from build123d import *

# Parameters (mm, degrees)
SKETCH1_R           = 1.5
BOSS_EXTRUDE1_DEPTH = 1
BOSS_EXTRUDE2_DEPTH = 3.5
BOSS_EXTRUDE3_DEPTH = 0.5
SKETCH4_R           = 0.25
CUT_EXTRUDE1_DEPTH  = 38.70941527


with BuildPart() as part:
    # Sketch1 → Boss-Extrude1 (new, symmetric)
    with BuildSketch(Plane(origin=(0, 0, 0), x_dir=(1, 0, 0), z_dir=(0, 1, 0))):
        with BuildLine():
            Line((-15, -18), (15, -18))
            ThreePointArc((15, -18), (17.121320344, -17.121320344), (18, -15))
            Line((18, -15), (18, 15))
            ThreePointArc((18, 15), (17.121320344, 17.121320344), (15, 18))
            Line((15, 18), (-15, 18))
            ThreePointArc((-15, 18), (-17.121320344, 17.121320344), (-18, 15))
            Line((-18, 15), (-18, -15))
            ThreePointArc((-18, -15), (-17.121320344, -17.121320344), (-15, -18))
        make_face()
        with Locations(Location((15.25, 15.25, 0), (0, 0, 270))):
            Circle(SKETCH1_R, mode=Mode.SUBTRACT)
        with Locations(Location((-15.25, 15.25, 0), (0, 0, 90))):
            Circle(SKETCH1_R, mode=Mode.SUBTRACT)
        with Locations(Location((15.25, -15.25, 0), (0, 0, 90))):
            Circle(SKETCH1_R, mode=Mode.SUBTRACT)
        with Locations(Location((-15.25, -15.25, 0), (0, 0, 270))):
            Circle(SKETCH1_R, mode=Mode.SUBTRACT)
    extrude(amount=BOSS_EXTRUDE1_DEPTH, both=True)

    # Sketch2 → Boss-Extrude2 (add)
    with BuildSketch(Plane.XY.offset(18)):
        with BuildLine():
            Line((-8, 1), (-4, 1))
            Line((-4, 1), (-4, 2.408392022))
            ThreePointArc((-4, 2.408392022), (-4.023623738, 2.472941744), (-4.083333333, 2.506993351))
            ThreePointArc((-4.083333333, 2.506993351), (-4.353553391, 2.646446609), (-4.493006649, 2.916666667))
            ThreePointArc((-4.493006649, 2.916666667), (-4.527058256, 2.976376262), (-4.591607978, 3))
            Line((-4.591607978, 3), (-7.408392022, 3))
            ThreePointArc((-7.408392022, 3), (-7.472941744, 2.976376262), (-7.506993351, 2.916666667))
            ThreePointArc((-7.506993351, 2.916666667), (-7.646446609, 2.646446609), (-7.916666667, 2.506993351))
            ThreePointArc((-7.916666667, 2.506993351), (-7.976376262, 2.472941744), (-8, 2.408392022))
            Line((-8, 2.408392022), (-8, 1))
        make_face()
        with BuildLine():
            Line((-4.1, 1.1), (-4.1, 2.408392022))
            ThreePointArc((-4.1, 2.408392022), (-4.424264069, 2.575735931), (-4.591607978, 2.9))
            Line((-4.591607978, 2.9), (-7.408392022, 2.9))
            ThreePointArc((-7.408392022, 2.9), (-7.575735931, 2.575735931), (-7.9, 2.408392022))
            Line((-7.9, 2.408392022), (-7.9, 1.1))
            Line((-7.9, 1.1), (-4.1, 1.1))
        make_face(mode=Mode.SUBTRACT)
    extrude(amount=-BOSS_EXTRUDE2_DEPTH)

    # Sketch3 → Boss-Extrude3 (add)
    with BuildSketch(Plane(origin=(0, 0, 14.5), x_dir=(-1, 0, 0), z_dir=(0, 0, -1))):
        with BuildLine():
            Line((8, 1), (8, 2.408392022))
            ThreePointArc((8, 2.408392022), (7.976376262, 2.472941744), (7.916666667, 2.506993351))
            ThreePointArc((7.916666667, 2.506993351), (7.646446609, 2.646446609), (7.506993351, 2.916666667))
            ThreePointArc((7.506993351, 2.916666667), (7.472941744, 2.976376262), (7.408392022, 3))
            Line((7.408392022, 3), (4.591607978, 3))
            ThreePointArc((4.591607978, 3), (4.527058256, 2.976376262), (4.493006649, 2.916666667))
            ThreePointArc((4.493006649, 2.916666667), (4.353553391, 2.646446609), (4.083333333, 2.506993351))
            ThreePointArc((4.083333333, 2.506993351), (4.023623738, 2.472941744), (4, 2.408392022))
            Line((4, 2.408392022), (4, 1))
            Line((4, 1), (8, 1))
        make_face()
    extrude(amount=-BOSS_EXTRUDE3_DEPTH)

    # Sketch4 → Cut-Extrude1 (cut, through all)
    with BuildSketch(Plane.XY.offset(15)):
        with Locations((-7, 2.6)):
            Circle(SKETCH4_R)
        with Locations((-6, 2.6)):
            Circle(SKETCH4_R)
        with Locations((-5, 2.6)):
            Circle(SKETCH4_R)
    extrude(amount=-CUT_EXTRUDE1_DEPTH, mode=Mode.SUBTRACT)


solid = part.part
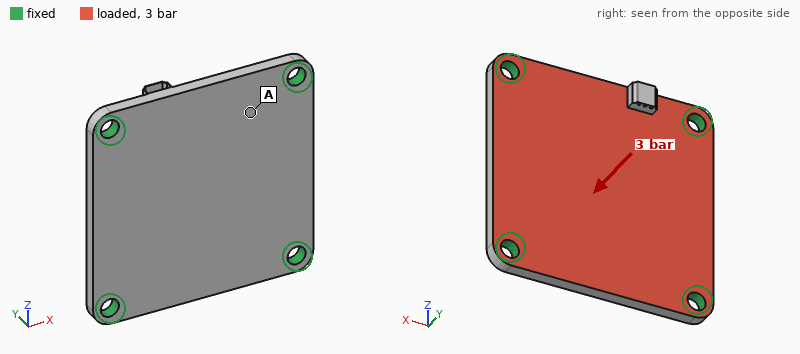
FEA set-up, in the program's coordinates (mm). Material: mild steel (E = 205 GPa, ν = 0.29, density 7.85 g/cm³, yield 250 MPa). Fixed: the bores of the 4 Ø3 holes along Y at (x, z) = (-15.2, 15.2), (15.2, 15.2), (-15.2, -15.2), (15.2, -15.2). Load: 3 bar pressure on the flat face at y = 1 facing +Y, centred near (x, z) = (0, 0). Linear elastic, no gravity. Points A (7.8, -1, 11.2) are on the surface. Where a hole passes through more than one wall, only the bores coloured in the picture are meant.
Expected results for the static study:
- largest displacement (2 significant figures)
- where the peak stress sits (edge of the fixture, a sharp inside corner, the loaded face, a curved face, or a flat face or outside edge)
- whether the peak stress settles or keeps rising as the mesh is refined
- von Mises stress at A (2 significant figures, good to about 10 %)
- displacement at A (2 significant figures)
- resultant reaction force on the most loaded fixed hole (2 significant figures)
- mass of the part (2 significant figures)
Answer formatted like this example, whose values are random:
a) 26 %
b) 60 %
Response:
a) 12 µm
b) edge of the fixture
c) keeps rising
d) 8.5 MPa
e) 5.3 µm
f) 95 N
g) 20 g
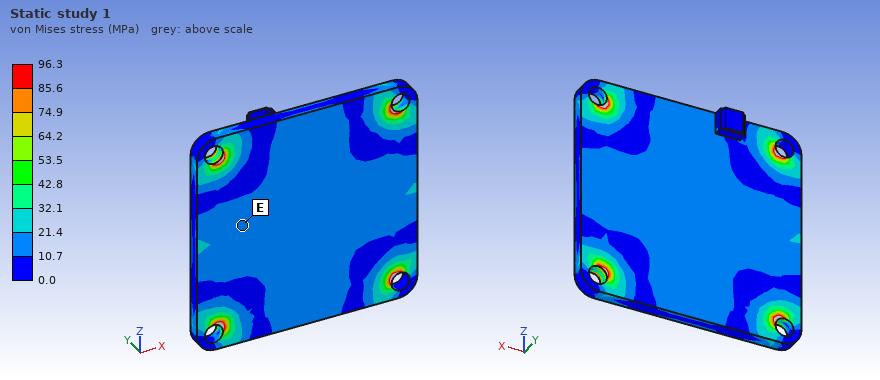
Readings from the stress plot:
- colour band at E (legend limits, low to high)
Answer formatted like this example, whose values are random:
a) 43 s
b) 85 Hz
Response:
a) 10.7 to 21.4 MPa
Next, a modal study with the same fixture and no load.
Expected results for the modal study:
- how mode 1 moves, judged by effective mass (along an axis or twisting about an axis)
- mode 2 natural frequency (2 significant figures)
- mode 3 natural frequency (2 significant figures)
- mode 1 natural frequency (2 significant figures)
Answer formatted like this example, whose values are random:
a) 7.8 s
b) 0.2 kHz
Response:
a) along Y
b) 13 kHz
c) 13 kHz
d) 7900 Hz
